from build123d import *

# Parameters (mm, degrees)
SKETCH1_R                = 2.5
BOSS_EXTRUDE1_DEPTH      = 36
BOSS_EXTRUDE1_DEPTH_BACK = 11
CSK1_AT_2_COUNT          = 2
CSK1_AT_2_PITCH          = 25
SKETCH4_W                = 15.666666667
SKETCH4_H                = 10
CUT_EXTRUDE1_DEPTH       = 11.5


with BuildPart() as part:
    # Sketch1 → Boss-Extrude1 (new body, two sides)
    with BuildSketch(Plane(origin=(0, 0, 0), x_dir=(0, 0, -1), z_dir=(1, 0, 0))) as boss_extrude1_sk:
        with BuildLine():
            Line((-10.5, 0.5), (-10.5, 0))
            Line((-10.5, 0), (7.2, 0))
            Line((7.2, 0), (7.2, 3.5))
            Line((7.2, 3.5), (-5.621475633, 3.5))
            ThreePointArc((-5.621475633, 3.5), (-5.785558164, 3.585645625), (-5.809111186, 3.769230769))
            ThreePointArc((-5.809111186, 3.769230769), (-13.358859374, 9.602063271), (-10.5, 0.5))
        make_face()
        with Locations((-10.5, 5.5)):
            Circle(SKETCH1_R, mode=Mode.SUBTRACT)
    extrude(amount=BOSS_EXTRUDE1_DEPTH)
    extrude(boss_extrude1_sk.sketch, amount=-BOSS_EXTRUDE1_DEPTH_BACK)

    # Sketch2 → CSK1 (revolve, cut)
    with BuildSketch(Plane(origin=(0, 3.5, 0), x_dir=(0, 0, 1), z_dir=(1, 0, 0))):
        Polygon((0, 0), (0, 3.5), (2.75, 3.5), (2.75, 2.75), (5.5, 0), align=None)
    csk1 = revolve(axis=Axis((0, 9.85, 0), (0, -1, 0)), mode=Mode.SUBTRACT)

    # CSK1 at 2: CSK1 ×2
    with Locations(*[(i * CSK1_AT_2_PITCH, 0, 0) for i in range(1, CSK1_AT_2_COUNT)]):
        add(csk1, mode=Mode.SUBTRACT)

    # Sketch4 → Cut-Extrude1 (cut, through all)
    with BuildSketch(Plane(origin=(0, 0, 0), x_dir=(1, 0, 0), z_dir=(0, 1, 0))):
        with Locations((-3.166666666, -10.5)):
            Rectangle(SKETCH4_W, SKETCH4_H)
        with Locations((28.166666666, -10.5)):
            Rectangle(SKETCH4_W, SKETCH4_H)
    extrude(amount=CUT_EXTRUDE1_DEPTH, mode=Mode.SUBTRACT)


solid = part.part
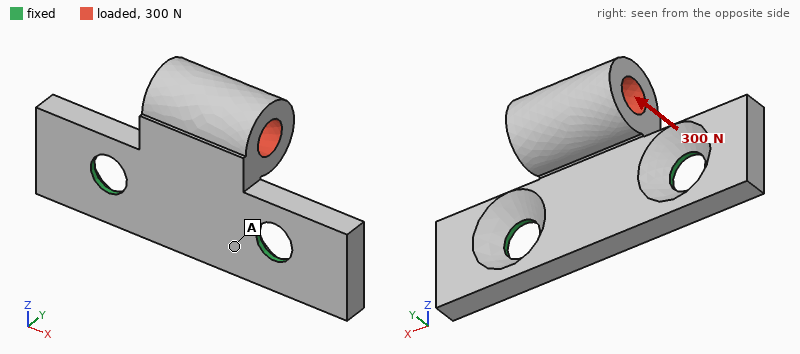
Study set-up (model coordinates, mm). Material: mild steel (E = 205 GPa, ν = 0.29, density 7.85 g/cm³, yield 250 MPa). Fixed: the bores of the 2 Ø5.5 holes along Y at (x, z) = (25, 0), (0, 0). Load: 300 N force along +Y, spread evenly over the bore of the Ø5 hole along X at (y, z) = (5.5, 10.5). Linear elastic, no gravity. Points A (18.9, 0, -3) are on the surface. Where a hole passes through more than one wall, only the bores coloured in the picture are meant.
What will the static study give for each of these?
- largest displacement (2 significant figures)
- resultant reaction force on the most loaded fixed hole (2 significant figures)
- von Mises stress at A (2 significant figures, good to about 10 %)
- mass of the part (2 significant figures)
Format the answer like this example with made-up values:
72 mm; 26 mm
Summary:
38 µm; 270 N; 30 MPa; 22 g
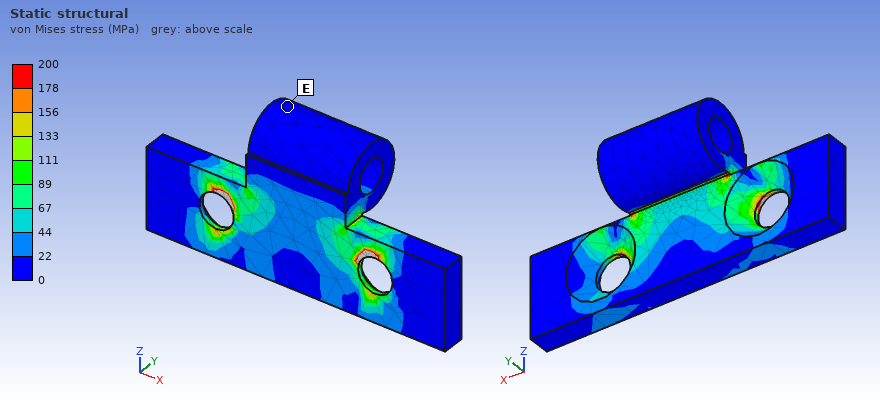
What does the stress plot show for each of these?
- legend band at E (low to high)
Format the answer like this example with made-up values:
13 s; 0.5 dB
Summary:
0 to 22 MPa
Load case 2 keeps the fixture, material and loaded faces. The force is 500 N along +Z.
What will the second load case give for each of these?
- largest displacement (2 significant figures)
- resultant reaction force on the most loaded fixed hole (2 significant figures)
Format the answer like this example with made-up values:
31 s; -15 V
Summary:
33 µm; 250 N
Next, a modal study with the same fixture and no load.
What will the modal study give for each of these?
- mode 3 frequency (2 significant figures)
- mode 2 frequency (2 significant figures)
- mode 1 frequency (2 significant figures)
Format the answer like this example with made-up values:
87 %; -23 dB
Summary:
15 kHz; 15 kHz; 5400 Hz
